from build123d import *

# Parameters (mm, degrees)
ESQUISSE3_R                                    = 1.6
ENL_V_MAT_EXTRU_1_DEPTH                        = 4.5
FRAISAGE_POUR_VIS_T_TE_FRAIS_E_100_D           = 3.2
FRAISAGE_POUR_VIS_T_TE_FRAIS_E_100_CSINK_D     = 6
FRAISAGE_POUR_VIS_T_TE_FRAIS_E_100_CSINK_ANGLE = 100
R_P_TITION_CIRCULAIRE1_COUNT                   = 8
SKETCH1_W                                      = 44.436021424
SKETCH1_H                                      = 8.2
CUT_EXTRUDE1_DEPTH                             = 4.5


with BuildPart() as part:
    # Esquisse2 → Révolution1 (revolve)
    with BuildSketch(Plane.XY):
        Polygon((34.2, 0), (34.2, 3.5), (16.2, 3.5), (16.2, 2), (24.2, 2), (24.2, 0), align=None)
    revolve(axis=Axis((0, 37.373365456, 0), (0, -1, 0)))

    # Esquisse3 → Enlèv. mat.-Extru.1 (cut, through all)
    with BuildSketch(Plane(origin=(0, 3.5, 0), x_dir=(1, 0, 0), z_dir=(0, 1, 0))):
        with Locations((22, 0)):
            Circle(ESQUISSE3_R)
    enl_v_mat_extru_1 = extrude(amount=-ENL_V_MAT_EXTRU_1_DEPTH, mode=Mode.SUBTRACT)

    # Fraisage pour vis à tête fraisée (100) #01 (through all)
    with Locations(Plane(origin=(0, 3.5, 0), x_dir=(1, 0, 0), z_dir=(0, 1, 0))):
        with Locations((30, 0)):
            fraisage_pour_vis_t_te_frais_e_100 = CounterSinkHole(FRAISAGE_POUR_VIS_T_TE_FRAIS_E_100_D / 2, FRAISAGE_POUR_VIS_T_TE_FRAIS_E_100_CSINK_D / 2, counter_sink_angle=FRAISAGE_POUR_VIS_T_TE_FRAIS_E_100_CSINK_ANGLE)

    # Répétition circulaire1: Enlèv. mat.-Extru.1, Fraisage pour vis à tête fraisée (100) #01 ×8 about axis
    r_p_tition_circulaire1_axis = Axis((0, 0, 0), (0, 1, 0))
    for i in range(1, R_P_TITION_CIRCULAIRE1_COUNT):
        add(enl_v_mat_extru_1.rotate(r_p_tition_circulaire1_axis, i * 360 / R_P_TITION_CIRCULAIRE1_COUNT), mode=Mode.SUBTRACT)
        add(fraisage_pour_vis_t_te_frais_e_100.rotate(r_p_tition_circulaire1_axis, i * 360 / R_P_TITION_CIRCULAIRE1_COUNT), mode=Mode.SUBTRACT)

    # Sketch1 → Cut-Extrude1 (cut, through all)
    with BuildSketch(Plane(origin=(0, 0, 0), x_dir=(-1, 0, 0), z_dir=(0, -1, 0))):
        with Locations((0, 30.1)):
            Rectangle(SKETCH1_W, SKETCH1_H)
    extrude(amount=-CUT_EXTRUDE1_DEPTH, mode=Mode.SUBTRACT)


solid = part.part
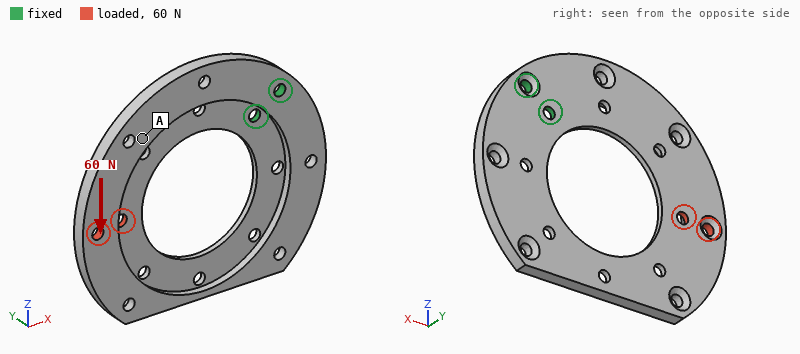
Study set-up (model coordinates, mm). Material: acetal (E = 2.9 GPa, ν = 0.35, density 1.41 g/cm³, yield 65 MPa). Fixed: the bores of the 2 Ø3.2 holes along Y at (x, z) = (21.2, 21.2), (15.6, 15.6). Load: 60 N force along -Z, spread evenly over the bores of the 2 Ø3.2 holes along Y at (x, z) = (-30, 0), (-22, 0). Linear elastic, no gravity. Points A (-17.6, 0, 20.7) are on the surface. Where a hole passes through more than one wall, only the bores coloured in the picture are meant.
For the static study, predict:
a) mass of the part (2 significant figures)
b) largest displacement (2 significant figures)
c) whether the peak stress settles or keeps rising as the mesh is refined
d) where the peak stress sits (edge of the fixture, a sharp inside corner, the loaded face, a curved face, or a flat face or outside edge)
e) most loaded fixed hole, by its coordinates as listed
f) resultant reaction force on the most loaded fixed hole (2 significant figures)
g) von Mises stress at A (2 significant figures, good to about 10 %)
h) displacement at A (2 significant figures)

9.5 g
0.98 mm
keeps rising
edge of the fixture
(15.6, 15.6)
270 N
3.2 MPa
0.74 mm
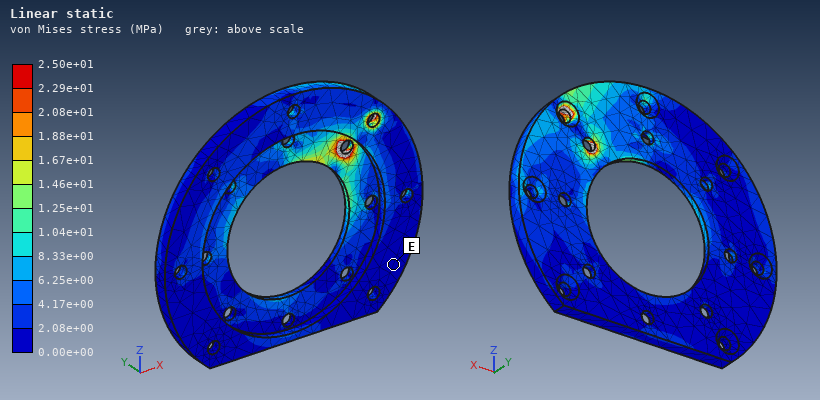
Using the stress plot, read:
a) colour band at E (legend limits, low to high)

0.00e+00 to 2.08e+00 MPa
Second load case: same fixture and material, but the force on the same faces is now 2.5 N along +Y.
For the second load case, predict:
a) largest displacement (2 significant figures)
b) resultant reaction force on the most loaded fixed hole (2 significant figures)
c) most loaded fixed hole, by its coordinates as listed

0.98 mm
12 N
(15.6, 15.6)
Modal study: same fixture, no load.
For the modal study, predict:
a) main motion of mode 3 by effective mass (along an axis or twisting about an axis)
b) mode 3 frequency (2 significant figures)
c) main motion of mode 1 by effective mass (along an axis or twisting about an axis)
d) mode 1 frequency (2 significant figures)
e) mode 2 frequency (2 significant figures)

along Y
560 Hz
along Y
150 Hz
290 Hz
